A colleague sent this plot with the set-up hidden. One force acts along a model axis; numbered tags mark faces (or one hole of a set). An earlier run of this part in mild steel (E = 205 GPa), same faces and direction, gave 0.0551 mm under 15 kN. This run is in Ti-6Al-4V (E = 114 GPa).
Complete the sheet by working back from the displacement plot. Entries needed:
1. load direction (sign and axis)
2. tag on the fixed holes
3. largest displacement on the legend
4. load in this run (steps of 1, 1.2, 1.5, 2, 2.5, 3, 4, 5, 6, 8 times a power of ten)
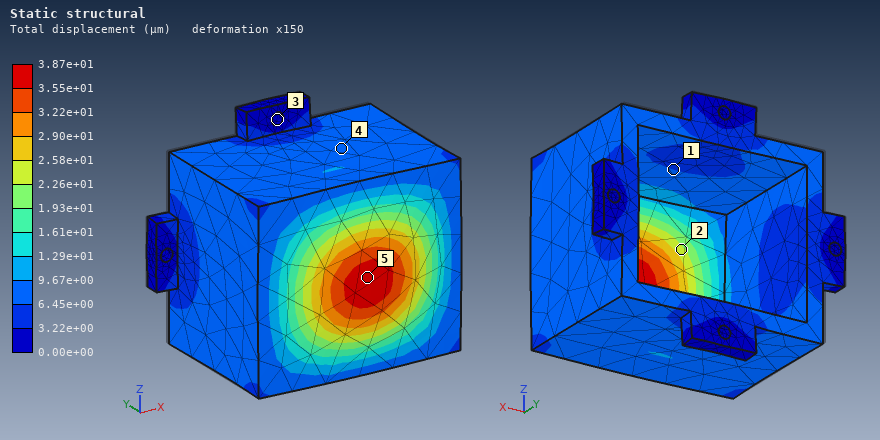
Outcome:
-Y
3
3.87e+01 µm
6 kN
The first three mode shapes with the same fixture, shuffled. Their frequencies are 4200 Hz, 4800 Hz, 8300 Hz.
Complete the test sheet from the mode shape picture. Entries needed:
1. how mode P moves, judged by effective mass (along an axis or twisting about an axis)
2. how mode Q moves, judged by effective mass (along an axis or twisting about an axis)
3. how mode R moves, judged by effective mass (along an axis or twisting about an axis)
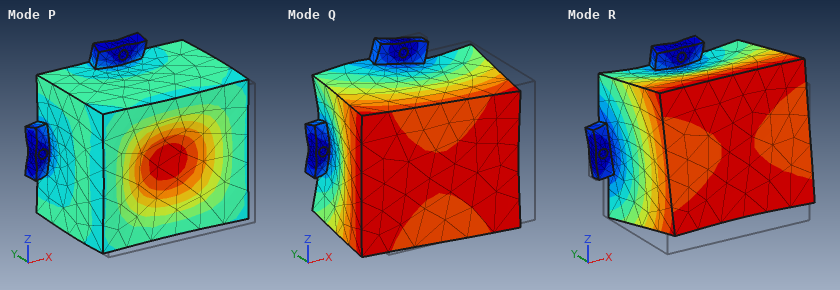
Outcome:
along Y
along X
along Z
